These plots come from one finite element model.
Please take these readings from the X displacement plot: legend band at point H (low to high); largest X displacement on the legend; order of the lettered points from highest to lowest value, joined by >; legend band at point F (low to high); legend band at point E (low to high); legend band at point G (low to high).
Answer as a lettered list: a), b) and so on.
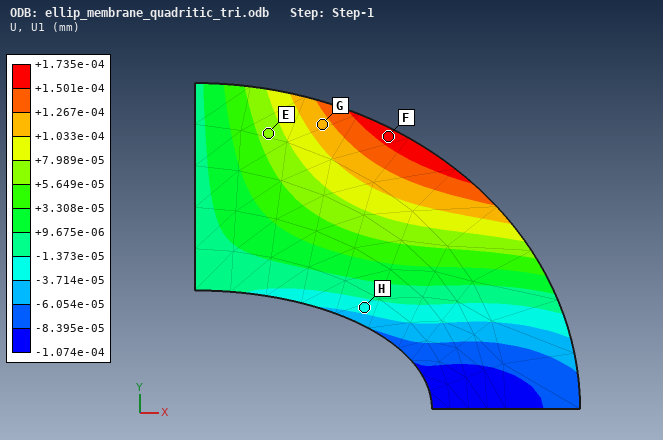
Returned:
a) -3.714e-05 to -1.373e-05 mm
b) +1.735e-04 mm
c) F > G > E > H
d) +1.501e-04 to +1.735e-04 mm
e) +5.649e-05 to +7.989e-05 mm
f) +1.033e-04 to +1.267e-04 mm
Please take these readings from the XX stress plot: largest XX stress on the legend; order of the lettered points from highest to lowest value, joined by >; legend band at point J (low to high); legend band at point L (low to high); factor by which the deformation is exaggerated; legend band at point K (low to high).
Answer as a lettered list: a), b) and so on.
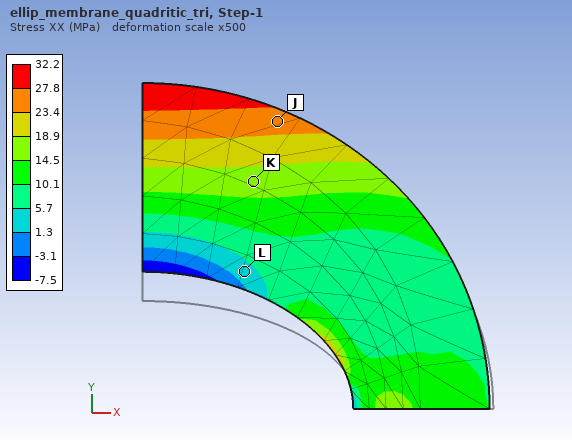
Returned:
a) 32.2 MPa
b) J > K > L
c) 23.4 to 27.8 MPa
d) 1.3 to 5.7 MPa
e) 500
f) 14.5 to 18.9 MPa
